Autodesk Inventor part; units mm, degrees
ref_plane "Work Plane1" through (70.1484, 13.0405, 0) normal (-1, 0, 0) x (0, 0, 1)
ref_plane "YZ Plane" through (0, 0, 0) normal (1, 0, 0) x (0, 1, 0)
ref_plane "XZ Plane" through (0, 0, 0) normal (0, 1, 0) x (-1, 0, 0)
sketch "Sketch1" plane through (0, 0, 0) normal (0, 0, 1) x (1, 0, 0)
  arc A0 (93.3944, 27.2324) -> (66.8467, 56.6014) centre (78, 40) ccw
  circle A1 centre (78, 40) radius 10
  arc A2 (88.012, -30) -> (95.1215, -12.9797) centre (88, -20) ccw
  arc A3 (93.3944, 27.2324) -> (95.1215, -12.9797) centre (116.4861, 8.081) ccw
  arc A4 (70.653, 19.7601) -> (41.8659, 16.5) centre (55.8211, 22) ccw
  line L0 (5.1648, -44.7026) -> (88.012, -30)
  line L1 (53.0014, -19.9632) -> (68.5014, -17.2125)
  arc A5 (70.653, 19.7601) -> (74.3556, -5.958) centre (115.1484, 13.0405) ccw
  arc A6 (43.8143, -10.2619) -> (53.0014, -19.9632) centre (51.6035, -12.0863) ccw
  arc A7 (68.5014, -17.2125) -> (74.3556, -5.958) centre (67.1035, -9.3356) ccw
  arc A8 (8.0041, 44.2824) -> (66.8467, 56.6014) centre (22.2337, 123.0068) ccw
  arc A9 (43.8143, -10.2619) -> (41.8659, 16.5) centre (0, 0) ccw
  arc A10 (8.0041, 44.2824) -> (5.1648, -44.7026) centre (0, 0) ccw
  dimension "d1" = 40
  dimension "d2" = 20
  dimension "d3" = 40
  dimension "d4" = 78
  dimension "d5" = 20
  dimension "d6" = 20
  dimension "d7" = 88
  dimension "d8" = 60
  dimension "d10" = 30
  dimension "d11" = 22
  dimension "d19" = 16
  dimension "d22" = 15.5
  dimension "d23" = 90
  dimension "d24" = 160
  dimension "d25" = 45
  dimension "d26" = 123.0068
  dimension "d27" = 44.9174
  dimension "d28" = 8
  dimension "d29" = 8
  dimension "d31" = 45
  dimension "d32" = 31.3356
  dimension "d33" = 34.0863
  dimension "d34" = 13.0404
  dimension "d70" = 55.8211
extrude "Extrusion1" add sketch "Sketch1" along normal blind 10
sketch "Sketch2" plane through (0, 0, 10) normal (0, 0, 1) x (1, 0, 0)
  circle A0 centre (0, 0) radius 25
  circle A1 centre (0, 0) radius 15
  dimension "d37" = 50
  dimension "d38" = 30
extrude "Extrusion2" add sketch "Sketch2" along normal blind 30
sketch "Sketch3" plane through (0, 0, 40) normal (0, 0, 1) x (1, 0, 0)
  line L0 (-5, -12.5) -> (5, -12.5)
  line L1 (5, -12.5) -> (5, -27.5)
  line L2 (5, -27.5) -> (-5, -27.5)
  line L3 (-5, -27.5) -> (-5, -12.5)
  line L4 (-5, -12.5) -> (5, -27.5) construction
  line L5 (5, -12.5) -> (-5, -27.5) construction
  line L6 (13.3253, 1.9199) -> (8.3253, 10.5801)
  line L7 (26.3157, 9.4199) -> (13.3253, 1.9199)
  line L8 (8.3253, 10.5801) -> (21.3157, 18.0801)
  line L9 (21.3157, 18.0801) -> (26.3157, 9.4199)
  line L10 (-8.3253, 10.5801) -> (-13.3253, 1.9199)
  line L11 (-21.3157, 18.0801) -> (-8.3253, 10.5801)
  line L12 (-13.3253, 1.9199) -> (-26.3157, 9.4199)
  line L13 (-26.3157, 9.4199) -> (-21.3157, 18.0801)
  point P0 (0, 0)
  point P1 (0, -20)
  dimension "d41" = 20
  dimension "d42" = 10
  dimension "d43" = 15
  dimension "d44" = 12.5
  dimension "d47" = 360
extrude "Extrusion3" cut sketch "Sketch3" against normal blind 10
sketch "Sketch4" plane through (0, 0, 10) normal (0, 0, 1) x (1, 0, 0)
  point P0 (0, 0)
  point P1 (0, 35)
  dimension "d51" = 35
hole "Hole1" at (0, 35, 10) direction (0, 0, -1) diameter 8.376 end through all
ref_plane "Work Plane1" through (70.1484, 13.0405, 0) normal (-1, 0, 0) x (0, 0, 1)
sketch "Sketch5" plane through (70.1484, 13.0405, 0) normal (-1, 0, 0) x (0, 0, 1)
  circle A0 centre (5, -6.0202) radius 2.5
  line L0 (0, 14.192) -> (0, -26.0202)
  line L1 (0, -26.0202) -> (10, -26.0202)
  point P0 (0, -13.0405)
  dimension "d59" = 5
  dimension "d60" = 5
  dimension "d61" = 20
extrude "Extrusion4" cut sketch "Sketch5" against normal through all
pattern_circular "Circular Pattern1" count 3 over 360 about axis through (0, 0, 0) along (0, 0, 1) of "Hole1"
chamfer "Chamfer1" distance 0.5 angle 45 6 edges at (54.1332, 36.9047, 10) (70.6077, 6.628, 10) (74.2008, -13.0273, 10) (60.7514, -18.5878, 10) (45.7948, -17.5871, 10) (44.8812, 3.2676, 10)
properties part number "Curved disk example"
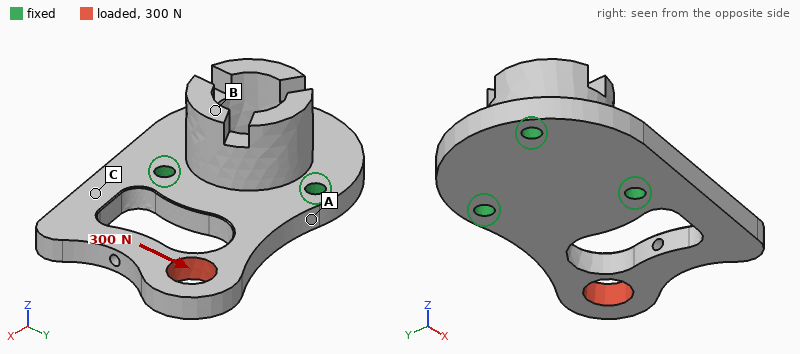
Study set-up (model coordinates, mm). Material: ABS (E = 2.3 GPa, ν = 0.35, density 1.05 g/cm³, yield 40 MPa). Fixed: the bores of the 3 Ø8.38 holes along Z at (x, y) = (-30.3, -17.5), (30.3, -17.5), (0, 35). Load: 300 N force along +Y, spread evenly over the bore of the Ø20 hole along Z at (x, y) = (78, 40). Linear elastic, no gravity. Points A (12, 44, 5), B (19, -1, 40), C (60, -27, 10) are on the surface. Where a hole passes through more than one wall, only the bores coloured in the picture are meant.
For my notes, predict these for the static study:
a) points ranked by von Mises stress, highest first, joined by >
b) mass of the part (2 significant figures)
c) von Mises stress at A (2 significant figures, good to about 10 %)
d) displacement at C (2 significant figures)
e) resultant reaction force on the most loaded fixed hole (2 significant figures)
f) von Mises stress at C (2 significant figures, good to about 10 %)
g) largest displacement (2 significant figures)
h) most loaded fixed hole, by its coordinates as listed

C > A > B
130 g
1.6 MPa
0.11 mm
360 N
2.6 MPa
0.34 mm
(30.3, -17.5)
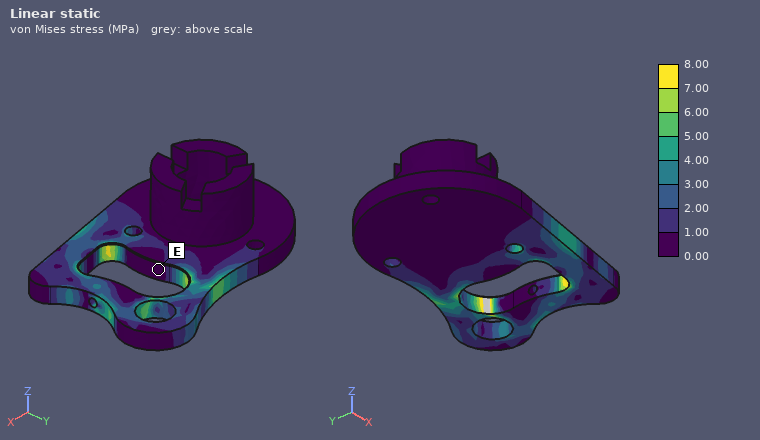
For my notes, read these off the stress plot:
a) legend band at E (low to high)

0.00 to 1.00 MPa
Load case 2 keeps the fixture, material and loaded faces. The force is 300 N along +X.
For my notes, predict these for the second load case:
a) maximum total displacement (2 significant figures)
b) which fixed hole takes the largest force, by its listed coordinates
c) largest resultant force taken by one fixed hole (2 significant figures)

0.16 mm
(0, 35)
270 N
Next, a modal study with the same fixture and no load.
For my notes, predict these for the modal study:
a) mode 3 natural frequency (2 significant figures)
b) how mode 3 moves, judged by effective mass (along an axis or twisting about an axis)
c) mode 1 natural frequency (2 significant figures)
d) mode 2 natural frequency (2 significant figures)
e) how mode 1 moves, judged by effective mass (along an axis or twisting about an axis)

1200 Hz
along Y
340 Hz
680 Hz
along Z
